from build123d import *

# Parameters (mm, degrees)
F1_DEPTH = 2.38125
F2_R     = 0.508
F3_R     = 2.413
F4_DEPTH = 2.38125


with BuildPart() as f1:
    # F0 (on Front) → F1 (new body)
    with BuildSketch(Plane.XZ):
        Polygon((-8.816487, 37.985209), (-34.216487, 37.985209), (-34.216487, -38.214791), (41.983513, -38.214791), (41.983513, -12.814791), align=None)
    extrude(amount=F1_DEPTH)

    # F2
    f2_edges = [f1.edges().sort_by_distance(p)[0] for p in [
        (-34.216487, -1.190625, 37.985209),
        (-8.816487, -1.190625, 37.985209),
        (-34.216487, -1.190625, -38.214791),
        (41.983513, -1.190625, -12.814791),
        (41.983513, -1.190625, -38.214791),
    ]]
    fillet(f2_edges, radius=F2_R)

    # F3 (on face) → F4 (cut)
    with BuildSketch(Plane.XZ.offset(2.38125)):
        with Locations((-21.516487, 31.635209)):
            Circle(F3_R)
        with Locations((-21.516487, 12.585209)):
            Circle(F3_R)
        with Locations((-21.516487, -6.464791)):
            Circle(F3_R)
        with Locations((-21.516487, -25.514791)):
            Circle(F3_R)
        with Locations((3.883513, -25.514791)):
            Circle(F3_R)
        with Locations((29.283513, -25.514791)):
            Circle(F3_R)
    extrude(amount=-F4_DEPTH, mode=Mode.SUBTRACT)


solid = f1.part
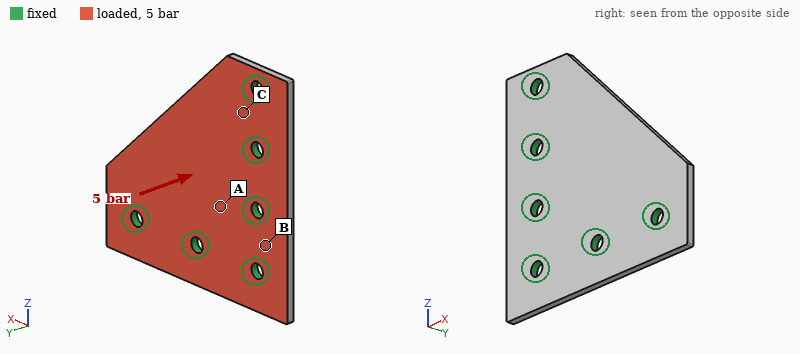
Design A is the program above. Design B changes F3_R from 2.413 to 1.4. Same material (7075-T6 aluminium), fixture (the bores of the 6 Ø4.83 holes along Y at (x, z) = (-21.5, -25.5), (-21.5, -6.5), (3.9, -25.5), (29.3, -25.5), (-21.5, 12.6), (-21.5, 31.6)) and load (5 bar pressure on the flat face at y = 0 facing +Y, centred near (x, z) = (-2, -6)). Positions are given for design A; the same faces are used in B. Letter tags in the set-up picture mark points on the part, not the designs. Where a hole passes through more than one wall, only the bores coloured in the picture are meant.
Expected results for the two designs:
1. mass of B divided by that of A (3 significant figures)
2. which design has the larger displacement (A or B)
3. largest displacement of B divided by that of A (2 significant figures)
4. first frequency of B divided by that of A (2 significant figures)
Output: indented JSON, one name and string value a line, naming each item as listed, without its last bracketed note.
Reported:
{
  "mass of B divided by that of A": "1.02",
  "which design has the larger displacement": "B",
  "largest displacement of B divided by that of A": "1.2",
  "first frequency of B divided by that of A": "0.91"
}
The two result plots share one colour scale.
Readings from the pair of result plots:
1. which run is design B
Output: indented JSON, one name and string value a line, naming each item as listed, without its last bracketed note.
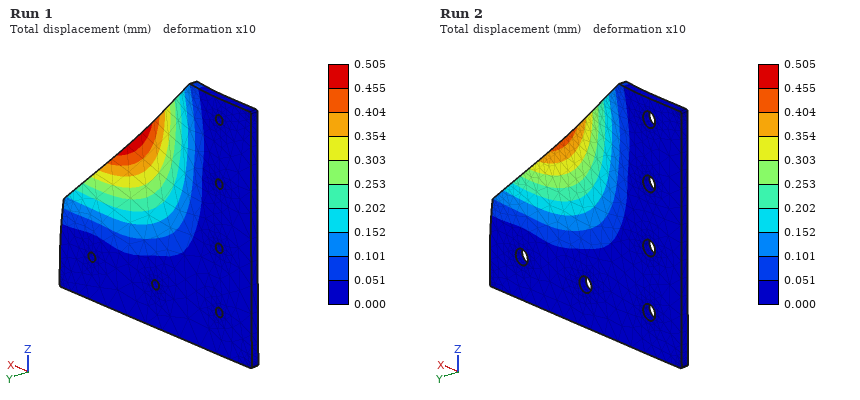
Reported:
{
  "which run is design B": "Run 1"
}
